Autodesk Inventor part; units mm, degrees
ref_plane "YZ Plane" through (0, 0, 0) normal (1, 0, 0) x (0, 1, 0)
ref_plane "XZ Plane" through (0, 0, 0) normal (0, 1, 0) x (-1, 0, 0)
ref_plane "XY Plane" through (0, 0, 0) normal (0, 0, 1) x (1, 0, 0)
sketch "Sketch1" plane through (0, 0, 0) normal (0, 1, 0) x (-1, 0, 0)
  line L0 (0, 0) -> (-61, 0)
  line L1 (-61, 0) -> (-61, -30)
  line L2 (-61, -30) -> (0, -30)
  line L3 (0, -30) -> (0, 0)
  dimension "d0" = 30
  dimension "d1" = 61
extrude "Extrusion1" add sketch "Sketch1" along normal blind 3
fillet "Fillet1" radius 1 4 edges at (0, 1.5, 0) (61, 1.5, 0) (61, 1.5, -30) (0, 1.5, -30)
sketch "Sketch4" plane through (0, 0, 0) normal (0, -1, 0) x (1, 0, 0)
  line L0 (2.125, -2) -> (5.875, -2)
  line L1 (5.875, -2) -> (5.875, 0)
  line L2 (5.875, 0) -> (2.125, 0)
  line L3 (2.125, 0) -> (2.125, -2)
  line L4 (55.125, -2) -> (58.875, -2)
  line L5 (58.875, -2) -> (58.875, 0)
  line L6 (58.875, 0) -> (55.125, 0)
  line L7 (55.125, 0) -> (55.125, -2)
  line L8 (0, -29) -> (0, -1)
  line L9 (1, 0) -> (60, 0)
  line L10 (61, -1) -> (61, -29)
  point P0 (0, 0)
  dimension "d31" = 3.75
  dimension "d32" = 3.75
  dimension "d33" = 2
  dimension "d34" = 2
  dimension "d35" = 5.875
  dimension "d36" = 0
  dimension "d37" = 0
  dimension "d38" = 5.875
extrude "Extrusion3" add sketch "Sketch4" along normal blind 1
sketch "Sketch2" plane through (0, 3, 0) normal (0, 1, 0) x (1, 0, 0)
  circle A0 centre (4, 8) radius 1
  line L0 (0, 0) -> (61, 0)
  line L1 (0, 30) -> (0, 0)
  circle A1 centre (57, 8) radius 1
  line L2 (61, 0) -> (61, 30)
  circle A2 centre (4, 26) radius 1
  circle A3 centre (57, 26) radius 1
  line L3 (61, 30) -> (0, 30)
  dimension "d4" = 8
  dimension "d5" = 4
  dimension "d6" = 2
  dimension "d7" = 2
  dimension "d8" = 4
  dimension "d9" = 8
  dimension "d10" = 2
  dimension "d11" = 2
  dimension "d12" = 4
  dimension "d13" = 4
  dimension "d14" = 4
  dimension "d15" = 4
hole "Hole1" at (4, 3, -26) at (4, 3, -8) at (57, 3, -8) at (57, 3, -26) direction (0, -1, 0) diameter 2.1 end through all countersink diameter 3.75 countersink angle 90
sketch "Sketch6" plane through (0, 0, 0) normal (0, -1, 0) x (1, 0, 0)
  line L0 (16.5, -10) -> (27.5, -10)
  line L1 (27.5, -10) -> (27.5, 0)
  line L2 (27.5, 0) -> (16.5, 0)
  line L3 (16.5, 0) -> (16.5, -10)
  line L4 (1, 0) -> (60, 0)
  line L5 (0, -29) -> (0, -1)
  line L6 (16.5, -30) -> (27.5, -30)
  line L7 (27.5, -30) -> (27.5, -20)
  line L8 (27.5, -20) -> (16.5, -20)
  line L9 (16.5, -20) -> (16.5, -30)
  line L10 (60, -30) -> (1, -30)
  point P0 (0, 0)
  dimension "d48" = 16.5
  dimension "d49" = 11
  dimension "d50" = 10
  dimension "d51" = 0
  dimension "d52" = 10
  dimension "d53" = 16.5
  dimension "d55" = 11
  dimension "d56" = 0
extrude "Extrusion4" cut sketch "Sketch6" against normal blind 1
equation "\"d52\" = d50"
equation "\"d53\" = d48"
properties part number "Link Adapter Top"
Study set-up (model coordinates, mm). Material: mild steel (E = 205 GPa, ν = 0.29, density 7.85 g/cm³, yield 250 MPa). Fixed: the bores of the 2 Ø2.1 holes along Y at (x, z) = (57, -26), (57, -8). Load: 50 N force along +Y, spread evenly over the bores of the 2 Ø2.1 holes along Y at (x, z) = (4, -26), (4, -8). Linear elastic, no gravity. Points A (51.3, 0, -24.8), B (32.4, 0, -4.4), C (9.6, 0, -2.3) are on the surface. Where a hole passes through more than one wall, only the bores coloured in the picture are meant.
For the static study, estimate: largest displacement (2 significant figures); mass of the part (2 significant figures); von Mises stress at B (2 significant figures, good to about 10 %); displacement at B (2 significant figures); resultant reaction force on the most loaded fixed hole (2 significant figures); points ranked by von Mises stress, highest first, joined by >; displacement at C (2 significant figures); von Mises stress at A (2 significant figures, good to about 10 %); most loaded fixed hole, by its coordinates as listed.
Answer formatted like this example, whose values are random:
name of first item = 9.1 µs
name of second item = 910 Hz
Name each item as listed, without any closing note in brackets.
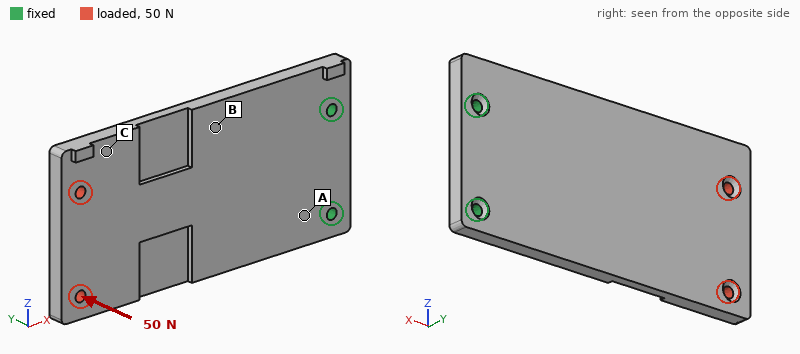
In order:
largest displacement = 0.25 mm
mass of the part = 41 g
von Mises stress at B = 28 MPa
displacement at B = 0.061 mm
resultant reaction force on the most loaded fixed hole = 30 N
points ranked by von Mises stress, highest first, joined by > = A > B > C
displacement at C = 0.18 mm
von Mises stress at A = 53 MPa
most loaded fixed hole, by its coordinates as listed = (57, -8)
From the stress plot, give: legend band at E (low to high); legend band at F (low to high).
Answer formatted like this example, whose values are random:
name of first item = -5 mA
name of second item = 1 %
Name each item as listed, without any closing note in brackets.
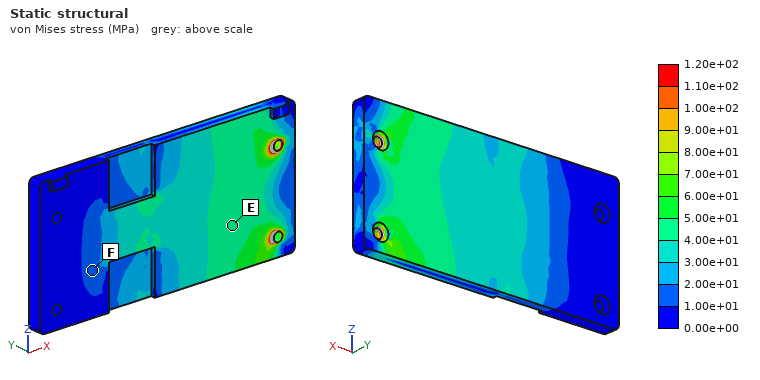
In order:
legend band at E = 4.00e+01 to 5.00e+01 MPa
legend band at F = 1.00e+01 to 2.00e+01 MPa
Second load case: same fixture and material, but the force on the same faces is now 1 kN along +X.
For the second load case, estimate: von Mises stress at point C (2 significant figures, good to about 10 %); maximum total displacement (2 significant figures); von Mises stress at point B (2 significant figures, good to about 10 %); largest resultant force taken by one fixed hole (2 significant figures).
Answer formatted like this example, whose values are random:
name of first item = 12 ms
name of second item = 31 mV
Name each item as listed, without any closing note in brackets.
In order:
von Mises stress at point C = 13 MPa
maximum total displacement = 67 µm
von Mises stress at point B = 15 MPa
largest resultant force taken by one fixed hole = 510 N
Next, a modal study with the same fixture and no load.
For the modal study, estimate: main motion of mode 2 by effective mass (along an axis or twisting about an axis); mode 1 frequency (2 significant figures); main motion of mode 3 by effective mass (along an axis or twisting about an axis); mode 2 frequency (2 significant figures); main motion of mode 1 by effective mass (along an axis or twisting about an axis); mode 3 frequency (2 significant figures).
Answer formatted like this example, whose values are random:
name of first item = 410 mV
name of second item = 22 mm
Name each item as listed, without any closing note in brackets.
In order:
main motion of mode 2 by effective mass = twisting about X
mode 1 frequency = 710 Hz
main motion of mode 3 by effective mass = along Y
mode 2 frequency = 2900 Hz
main motion of mode 1 by effective mass = along Y
mode 3 frequency = 4000 Hz
